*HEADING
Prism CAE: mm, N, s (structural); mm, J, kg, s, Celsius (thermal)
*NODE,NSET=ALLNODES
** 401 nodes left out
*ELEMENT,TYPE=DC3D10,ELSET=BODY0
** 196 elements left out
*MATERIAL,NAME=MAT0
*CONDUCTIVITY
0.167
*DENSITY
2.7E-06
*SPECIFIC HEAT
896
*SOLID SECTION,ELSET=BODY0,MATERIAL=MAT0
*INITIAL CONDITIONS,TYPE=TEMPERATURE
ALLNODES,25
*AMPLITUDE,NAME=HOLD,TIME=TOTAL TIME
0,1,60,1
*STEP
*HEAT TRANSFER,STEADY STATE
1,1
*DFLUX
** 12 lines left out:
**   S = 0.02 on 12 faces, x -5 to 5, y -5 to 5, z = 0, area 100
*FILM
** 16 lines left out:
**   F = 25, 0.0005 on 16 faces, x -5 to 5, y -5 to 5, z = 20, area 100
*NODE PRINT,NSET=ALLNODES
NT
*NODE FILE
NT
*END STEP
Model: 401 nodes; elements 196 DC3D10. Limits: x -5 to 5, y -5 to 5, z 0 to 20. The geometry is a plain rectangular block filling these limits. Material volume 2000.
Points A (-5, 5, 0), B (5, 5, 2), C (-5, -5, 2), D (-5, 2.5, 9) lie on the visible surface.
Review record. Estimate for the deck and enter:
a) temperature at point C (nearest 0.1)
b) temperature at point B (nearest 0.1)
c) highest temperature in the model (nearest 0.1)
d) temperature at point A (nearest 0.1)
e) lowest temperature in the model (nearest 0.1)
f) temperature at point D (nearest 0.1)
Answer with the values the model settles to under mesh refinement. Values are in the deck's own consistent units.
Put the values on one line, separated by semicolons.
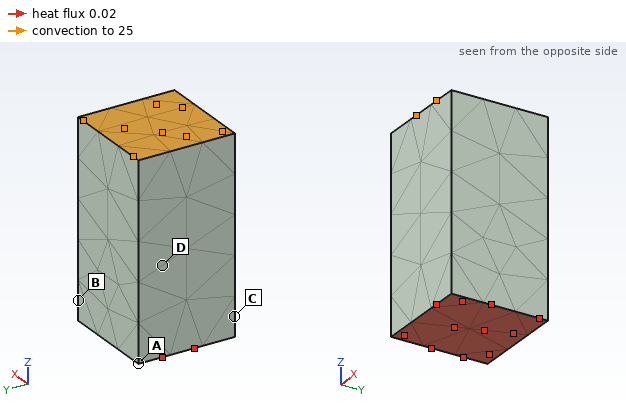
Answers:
67.2; 67.2; 67.4; 67.4; 65.0; 66.3
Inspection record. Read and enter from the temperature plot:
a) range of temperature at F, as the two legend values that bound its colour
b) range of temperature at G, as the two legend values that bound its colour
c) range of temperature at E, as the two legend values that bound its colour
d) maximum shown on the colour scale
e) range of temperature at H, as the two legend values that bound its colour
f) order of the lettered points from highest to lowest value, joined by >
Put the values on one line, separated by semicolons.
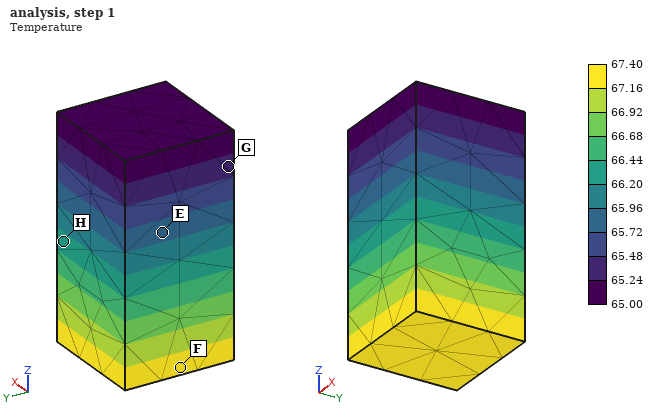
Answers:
67.16 to 67.40; 65.24 to 65.48; 65.72 to 65.96; 67.40; 66.20 to 66.44; F > H > E > G
